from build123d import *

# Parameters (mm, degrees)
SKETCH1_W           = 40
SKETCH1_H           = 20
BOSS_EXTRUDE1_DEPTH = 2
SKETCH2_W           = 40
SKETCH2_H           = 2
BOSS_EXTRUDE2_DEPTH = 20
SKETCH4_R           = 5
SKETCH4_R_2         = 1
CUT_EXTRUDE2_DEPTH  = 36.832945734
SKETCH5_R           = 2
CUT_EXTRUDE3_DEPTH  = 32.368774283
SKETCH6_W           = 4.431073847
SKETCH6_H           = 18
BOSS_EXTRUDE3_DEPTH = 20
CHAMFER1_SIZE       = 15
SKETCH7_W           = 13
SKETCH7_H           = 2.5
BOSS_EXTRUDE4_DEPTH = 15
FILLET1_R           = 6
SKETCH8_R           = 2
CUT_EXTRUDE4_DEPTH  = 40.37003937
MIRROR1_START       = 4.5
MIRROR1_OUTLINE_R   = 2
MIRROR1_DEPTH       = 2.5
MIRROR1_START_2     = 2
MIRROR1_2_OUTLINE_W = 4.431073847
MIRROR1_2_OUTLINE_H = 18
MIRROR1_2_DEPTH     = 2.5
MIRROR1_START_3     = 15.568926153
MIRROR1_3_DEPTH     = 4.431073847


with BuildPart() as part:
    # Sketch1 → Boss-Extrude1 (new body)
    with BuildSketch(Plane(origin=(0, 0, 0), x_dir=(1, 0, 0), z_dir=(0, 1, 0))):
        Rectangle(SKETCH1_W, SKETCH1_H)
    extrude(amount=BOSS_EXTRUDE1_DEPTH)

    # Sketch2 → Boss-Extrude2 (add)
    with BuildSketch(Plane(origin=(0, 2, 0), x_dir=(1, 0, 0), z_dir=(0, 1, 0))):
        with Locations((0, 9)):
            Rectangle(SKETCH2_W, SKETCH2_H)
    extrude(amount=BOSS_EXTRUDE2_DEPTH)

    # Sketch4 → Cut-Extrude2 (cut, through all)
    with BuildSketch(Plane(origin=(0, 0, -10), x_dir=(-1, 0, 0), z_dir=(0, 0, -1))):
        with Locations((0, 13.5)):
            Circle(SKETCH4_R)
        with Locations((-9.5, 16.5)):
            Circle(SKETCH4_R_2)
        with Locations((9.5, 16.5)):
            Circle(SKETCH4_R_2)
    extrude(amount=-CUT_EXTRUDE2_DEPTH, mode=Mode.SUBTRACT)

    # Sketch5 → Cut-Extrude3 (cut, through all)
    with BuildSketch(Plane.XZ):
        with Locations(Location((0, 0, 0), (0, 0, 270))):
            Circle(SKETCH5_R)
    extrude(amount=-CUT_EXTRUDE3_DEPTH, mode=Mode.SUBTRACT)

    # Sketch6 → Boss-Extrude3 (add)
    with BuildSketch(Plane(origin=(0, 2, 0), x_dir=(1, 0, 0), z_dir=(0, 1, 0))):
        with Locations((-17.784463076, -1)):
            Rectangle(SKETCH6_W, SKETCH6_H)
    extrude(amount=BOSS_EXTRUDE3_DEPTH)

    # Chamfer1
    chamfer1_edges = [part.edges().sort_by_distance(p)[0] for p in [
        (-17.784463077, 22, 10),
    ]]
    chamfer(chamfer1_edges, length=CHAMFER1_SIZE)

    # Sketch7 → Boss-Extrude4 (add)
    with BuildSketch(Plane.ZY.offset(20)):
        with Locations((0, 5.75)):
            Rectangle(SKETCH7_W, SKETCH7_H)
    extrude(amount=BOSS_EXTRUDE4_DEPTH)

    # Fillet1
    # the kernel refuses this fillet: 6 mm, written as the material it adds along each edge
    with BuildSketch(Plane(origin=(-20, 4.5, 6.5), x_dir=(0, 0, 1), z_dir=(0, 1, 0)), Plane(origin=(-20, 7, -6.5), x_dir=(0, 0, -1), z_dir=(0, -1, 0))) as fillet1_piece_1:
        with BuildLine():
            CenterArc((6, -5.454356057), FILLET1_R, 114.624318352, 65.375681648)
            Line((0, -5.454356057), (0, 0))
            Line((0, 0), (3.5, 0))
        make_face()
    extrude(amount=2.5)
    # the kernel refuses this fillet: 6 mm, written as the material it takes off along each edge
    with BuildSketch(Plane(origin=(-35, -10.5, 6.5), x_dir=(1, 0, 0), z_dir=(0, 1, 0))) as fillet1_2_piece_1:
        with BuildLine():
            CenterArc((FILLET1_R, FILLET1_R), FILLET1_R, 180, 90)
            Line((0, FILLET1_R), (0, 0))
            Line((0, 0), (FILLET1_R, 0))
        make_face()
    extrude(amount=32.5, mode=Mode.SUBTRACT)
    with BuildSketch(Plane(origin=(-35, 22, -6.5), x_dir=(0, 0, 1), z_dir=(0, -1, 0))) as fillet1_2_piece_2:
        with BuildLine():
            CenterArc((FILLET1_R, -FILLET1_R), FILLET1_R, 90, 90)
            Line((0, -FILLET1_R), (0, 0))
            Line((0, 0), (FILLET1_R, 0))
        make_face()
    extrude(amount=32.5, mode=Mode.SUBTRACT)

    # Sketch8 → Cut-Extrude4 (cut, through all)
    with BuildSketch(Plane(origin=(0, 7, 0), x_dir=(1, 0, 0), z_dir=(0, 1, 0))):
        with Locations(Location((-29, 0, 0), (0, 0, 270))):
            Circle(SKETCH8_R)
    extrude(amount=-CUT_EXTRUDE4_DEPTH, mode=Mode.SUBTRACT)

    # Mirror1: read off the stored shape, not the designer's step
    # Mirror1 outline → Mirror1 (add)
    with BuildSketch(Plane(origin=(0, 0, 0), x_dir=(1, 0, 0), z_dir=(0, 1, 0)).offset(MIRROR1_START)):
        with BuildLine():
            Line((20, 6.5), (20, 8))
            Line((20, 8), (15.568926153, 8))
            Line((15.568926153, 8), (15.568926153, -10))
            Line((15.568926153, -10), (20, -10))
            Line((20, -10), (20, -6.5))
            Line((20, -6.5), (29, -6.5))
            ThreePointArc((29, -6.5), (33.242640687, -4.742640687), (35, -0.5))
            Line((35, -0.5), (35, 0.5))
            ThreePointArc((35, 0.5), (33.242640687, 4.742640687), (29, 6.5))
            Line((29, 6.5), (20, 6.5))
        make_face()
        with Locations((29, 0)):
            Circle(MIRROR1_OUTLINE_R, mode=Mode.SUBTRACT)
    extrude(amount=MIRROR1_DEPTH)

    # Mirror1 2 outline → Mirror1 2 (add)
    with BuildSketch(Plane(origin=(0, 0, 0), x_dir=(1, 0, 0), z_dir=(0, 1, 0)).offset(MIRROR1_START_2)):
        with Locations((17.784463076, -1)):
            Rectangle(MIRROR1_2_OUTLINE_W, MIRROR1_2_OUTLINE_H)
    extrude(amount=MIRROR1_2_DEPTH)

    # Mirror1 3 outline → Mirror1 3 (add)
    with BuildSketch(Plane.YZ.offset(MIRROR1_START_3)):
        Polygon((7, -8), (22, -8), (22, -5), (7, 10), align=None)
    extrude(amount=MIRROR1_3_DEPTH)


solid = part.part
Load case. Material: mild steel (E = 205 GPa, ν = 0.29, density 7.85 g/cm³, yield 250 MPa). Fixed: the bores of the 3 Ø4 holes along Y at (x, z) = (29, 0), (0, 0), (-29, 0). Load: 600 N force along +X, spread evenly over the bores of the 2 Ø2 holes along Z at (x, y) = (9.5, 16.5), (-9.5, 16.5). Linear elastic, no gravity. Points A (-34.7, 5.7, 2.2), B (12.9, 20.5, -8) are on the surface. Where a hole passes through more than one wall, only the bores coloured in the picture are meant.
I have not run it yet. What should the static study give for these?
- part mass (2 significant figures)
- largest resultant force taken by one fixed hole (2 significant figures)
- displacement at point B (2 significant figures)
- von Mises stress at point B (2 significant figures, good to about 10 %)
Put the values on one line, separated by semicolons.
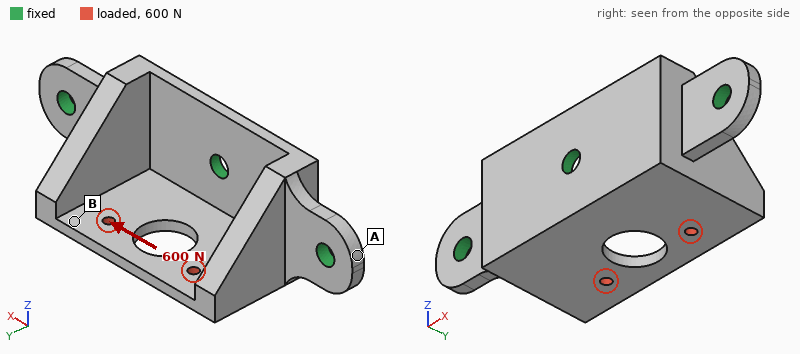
48 g; 400 N; 16 µm; 31 MPa
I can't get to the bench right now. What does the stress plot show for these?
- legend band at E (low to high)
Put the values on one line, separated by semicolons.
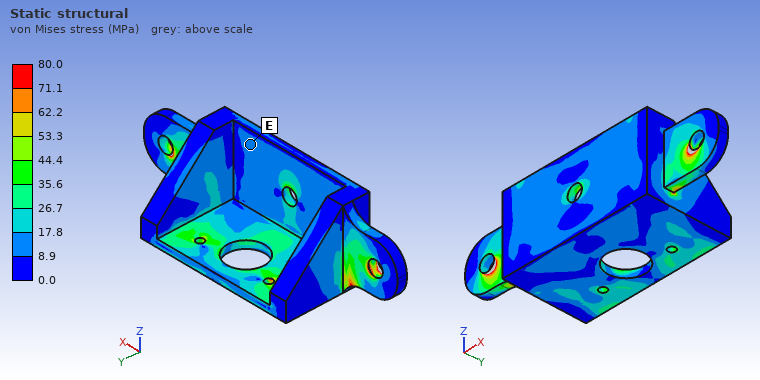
8.9 to 17.8 MPa
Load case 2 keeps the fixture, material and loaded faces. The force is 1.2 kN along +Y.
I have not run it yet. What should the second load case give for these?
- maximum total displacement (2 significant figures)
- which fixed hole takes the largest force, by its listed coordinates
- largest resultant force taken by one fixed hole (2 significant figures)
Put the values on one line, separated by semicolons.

55 µm; (0, 0); 970 N
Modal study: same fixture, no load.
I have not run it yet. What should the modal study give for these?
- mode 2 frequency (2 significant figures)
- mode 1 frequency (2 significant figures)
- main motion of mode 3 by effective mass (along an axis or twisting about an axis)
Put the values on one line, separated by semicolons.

6300 Hz; 5300 Hz; along Y
